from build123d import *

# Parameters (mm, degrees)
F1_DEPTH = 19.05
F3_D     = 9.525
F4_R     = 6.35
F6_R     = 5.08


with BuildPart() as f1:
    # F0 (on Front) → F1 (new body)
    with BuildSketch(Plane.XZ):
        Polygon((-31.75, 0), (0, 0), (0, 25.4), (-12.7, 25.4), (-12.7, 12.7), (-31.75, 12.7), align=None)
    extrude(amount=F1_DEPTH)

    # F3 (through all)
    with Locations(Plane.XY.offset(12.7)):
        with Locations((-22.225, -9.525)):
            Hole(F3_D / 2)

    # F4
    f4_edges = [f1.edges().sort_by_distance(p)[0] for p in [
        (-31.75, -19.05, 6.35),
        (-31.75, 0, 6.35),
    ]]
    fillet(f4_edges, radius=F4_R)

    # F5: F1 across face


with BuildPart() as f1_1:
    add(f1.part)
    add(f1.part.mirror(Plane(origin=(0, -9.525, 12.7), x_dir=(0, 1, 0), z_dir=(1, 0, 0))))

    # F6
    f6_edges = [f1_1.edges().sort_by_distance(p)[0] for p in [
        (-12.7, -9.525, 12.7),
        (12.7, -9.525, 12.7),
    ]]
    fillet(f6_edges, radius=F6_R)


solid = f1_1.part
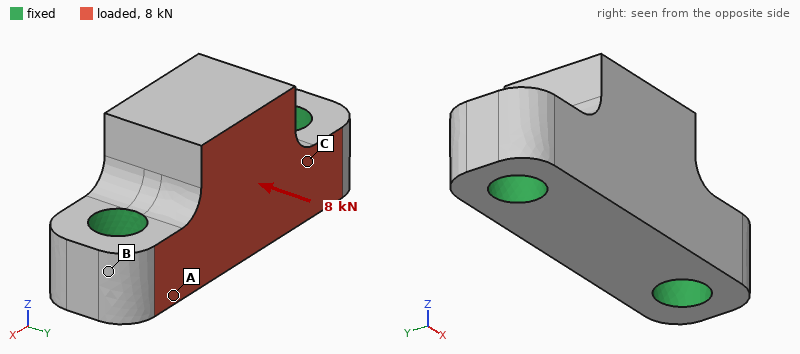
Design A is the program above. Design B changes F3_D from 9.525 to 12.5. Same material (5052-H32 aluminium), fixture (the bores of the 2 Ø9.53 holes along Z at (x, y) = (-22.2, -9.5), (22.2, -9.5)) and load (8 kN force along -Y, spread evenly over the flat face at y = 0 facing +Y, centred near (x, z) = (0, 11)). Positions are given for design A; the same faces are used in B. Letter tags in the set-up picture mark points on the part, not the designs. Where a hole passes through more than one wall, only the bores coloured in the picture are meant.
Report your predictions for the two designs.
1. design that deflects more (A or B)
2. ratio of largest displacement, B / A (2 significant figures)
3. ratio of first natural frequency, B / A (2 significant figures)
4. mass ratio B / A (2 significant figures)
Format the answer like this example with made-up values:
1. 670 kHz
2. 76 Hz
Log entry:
1. A
2. 0.79
3. 1.1
4. 0.93
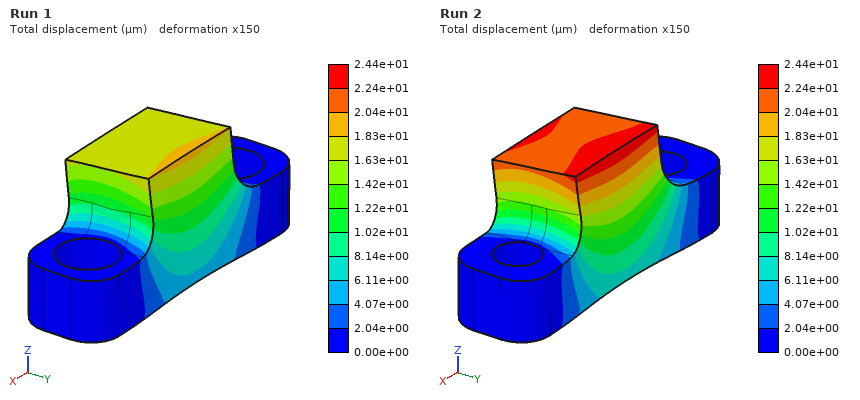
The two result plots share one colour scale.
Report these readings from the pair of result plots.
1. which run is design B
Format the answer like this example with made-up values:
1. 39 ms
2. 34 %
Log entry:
1. Run 1
